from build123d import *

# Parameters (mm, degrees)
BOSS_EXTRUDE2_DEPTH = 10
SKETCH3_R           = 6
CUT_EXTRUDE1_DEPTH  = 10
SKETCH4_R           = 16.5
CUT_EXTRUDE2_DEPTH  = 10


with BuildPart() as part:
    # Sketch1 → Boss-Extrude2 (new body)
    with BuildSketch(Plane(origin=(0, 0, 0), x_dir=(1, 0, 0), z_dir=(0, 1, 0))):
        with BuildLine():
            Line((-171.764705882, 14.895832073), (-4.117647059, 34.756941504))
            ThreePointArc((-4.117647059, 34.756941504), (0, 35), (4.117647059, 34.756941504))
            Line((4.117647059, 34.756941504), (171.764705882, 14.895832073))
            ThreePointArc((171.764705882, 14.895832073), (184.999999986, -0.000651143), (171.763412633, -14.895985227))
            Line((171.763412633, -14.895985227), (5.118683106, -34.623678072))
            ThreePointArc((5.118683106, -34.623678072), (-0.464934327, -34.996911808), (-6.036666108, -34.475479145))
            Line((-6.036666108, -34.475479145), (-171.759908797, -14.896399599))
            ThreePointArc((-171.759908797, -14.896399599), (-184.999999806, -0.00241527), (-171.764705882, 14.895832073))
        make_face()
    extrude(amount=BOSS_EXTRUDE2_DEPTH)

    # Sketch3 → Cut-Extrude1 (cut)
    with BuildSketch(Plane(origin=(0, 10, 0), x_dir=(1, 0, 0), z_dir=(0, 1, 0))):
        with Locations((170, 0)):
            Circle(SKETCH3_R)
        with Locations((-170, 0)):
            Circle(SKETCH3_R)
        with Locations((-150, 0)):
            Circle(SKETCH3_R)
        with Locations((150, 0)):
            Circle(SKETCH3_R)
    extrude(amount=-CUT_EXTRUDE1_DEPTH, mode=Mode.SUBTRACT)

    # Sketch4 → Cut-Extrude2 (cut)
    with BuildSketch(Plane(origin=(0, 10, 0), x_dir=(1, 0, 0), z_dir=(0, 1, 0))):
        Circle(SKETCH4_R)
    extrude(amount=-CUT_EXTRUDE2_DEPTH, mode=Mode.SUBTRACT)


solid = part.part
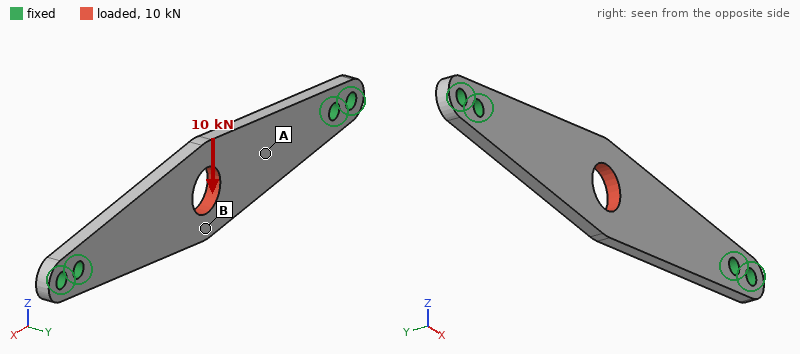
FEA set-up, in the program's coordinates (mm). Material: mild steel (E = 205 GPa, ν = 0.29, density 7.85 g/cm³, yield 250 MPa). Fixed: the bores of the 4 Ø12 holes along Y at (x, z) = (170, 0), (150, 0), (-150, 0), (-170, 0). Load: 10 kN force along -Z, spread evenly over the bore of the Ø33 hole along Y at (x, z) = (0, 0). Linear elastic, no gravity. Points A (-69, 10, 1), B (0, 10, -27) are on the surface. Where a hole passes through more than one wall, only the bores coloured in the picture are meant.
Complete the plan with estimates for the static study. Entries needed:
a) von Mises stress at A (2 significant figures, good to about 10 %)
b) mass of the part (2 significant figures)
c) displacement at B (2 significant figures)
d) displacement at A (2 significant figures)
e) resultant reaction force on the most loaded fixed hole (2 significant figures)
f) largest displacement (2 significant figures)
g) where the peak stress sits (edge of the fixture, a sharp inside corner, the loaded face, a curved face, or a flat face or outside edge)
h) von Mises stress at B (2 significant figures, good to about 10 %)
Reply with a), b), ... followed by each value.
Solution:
a) 20 MPa
b) 1.3 kg
c) 92 µm
d) 65 µm
e) 8.8 kN
f) 93 µm
g) edge of the fixture
h) 53 MPa
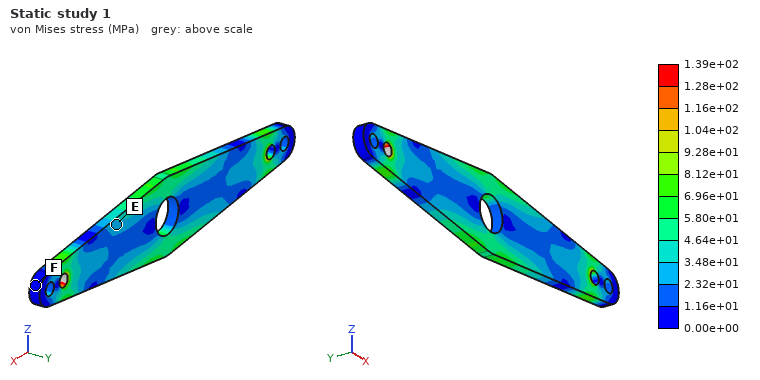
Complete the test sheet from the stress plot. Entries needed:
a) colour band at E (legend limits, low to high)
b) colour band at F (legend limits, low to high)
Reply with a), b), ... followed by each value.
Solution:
a) 2.32e+01 to 3.48e+01 MPa
b) 0.00e+00 to 1.16e+01 MPa
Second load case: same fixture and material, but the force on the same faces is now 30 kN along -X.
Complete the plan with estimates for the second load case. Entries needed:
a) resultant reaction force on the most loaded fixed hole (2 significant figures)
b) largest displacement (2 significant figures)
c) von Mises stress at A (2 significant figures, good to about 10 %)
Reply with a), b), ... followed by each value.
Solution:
a) 13 kN
b) 23 µm
c) 28 MPa
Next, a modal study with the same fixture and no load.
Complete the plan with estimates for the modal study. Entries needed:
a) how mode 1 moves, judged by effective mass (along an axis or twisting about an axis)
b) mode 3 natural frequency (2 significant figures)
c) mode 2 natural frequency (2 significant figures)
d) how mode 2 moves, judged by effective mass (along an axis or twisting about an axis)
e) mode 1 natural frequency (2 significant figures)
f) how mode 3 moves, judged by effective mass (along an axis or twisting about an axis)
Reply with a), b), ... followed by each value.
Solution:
a) along Y
b) 1600 Hz
c) 1500 Hz
d) twisting about X
e) 530 Hz
f) twisting about Z
